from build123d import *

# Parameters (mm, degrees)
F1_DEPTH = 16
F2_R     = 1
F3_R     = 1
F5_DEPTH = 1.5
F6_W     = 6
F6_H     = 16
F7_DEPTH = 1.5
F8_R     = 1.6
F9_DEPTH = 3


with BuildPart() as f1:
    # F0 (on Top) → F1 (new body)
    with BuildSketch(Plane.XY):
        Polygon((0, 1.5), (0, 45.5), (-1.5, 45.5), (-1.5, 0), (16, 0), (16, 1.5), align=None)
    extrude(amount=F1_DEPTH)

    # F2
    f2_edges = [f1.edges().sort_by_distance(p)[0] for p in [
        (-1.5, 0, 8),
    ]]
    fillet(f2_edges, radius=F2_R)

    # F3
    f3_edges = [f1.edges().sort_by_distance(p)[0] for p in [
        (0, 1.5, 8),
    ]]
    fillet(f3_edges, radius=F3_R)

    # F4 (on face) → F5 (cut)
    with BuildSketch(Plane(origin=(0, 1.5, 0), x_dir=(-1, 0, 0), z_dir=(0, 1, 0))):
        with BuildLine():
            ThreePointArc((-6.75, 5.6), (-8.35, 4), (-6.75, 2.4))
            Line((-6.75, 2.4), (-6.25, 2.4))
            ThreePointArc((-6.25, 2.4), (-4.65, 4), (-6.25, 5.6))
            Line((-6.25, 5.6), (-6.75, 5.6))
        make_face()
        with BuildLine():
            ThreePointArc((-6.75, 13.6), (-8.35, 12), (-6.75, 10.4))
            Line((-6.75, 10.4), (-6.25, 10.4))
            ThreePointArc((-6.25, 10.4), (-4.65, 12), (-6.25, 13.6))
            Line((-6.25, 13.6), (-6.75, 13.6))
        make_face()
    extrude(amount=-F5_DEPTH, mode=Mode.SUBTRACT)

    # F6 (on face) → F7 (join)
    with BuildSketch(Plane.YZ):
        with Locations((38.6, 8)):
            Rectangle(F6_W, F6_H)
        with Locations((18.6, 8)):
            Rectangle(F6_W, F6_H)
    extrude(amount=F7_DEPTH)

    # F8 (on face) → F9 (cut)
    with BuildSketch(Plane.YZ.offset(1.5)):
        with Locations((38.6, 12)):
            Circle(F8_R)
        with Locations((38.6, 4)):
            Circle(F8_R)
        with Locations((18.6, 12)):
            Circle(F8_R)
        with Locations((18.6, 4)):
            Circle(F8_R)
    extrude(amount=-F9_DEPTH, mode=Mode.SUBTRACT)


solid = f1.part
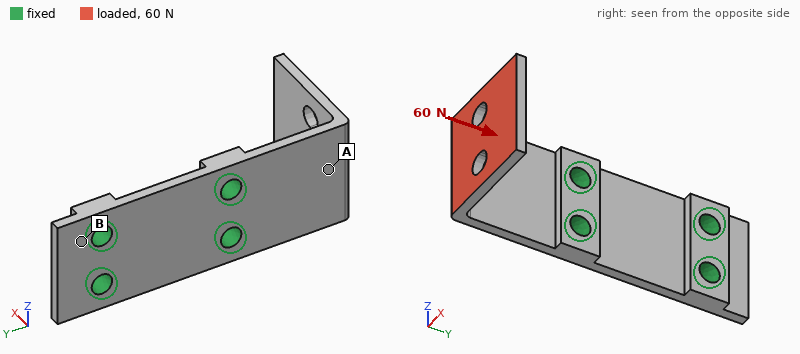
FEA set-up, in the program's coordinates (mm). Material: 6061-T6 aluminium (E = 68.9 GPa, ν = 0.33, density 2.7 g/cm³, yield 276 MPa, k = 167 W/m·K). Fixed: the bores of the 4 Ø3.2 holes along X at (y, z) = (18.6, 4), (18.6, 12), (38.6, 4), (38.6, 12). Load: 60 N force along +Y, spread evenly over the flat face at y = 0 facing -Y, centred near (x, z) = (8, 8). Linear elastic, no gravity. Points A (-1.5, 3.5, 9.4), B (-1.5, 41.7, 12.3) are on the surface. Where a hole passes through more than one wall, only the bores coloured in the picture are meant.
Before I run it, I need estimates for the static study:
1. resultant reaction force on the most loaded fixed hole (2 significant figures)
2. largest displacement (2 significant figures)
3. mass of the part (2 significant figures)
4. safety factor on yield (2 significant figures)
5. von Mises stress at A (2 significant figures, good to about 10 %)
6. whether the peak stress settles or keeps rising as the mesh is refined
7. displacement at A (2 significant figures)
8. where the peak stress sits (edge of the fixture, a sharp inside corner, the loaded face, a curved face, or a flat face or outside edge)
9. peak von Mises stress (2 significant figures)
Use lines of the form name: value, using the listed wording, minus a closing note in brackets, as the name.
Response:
resultant reaction force on the most loaded fixed hole: 31 N
largest displacement: 0.55 mm
mass of the part: 4.4 g
safety factor on yield: 2.7
von Mises stress at A: 77 MPa
whether the peak stress settles or keeps rising as the mesh is refined: settles
displacement at A: 0.13 mm
where the peak stress sits: a curved face
peak von Mises stress: 100 MPa
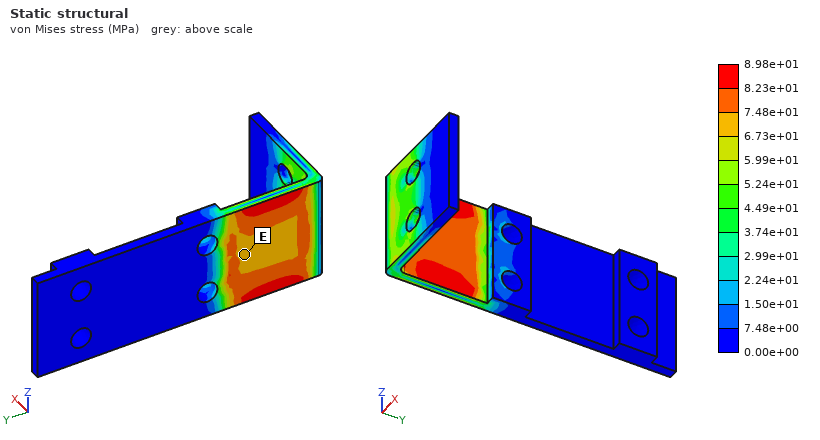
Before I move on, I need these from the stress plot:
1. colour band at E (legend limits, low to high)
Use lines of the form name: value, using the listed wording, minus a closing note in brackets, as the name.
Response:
colour band at E: 6.73e+01 to 7.48e+01 MPa
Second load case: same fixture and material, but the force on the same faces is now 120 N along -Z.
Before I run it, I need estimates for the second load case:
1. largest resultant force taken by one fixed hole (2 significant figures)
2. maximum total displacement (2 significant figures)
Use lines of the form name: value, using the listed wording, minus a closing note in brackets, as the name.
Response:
largest resultant force taken by one fixed hole: 220 N
maximum total displacement: 0.43 mm
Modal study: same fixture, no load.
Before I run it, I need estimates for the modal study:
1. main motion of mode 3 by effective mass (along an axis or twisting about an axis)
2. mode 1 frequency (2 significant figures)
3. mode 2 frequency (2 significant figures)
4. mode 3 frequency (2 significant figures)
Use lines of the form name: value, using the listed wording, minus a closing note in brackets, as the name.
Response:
main motion of mode 3 by effective mass: along X
mode 1 frequency: 1700 Hz
mode 2 frequency: 3000 Hz
mode 3 frequency: 4600 Hz
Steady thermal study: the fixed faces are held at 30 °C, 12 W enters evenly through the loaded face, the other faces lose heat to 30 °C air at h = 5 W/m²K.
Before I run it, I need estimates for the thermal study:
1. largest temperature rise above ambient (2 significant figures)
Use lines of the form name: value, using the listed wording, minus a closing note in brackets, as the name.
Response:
largest temperature rise above ambient: 75 K
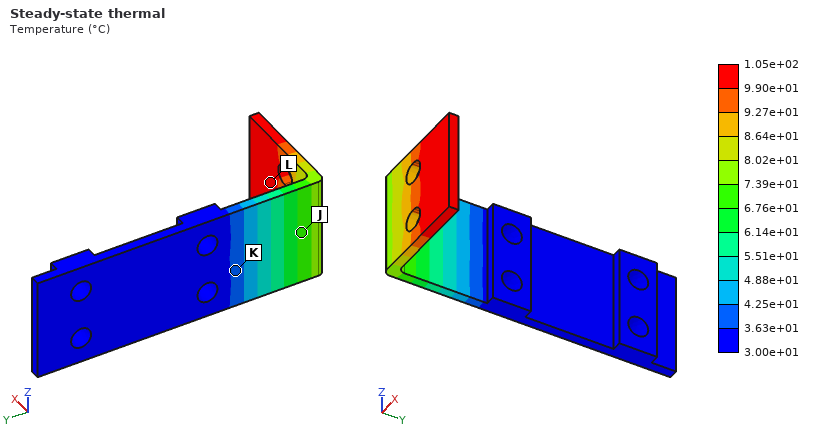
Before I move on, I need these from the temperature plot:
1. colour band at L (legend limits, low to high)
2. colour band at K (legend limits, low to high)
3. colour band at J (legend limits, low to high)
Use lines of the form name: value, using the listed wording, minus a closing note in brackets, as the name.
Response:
colour band at L: 9.90e+01 to 1.05e+02 °C
colour band at K: 3.63e+01 to 4.25e+01 °C
colour band at J: 6.76e+01 to 7.39e+01 °C
